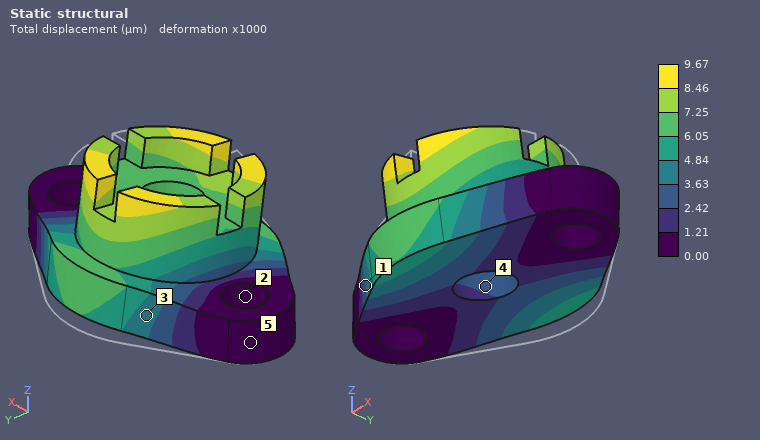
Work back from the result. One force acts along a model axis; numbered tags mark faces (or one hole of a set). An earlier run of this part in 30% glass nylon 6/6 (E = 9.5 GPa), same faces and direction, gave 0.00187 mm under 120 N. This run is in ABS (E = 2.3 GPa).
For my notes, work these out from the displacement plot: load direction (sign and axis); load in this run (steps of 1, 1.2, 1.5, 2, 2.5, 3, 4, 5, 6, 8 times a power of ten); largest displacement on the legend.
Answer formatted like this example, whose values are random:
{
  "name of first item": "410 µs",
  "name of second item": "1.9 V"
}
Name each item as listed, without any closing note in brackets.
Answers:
{
  "load direction": "-Y",
  "load in this run": "150 N",
  "largest displacement on the legend": "9.67 µm"
}
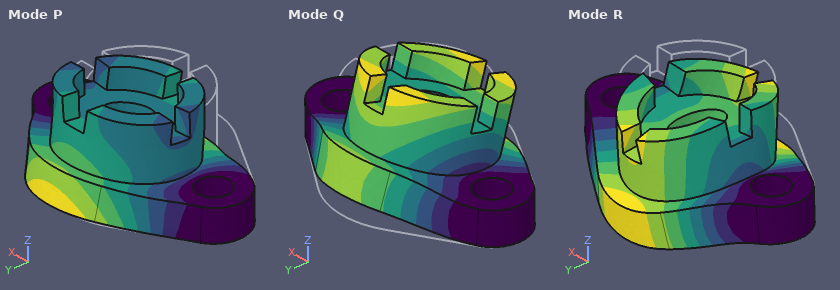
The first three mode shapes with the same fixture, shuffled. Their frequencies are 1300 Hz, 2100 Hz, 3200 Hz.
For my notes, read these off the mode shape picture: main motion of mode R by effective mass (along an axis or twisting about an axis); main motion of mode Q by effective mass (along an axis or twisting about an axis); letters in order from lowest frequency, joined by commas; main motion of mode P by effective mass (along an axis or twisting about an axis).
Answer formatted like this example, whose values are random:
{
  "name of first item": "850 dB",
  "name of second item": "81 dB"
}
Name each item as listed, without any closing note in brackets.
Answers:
{
  "main motion of mode R by effective mass": "along Z",
  "main motion of mode Q by effective mass": "along Y",
  "letters in order from lowest frequency, joined by commas": "Q, R, P",
  "main motion of mode P by effective mass": "along Y"
}
